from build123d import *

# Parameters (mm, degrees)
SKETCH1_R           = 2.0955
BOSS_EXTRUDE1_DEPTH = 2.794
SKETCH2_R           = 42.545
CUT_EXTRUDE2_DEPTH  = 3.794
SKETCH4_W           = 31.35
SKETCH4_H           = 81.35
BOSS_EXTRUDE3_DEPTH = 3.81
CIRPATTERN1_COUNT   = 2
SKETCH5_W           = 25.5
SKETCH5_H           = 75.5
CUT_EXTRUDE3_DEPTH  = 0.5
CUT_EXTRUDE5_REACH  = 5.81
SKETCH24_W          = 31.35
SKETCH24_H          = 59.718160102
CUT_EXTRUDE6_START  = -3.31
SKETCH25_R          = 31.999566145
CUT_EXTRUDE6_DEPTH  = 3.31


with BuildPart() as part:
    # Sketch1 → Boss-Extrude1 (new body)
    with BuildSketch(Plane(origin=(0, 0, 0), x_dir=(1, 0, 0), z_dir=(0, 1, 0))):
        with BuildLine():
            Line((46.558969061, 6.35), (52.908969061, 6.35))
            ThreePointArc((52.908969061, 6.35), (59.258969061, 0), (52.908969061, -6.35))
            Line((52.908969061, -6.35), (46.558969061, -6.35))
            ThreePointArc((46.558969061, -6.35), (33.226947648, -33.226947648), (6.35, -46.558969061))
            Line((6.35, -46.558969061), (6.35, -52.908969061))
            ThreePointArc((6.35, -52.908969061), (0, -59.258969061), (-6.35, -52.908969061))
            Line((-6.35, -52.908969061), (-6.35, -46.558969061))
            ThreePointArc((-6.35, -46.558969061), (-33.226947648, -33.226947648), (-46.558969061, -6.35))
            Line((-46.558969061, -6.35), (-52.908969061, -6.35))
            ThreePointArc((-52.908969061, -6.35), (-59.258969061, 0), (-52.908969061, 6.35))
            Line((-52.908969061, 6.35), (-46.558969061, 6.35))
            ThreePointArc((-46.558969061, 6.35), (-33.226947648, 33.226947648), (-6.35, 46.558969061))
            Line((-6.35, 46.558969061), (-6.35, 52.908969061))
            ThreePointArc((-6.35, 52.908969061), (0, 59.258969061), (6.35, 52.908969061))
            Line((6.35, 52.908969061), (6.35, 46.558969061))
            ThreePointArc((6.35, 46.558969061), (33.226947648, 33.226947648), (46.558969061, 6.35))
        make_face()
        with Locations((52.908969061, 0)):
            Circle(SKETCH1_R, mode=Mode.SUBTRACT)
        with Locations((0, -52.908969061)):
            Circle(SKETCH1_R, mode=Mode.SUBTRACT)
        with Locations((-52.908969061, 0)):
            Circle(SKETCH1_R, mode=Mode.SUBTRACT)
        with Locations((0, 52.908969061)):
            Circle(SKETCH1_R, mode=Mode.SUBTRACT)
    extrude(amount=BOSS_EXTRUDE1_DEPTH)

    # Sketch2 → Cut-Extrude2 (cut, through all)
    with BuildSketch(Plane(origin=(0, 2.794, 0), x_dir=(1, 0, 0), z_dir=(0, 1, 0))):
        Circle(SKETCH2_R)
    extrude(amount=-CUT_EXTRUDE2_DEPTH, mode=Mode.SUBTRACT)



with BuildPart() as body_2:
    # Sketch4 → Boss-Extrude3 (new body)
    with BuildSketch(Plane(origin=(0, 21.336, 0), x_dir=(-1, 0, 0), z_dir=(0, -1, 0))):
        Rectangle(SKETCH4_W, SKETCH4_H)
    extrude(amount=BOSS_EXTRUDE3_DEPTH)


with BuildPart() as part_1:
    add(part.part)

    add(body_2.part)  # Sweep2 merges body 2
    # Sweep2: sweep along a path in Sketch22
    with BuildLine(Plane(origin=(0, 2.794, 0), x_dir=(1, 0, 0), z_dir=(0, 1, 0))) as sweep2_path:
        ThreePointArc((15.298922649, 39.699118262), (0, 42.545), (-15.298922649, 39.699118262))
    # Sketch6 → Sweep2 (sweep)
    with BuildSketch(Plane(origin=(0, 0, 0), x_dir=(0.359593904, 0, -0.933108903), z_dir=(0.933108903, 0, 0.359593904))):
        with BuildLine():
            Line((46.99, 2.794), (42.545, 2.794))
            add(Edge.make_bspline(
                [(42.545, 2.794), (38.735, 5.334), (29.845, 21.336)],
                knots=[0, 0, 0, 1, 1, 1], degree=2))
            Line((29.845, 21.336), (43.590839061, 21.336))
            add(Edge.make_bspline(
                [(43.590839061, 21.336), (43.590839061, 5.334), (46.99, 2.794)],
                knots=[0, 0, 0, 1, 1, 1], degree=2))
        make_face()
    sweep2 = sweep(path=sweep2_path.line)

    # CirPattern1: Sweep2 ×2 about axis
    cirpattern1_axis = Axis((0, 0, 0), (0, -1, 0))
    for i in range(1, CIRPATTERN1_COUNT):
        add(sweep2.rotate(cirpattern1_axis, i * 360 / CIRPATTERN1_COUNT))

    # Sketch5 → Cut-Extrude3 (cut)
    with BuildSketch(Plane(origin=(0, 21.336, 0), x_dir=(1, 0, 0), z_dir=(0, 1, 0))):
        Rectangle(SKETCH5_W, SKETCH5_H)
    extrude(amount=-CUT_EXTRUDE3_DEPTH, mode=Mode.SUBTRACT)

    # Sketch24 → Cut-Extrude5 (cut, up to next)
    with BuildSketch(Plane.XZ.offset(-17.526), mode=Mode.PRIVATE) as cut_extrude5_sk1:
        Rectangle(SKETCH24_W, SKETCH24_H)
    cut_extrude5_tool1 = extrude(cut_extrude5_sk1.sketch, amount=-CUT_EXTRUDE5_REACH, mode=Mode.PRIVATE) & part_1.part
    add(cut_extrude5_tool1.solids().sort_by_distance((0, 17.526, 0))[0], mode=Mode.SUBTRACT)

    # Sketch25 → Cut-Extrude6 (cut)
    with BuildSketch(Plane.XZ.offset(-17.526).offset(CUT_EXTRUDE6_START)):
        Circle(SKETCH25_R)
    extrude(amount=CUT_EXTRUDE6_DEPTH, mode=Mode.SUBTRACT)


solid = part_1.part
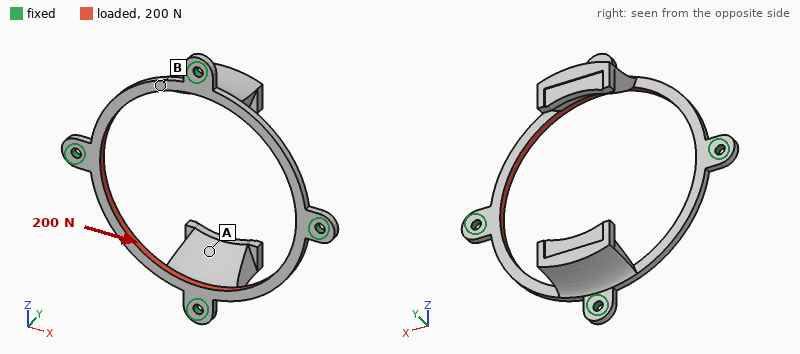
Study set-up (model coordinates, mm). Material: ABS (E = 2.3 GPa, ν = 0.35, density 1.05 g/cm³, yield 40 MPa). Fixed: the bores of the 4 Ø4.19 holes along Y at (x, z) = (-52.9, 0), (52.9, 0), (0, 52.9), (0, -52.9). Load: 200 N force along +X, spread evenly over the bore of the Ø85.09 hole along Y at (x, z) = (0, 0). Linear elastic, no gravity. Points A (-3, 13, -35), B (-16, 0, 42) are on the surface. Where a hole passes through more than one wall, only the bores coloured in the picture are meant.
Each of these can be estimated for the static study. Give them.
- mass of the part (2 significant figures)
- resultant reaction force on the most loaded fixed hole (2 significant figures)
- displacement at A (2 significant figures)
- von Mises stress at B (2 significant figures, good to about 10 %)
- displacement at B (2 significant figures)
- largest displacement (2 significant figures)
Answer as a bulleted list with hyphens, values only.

- 15 g
- 81 N
- 0.073 mm
- 2.7 MPa
- 0.066 mm
- 0.11 mm
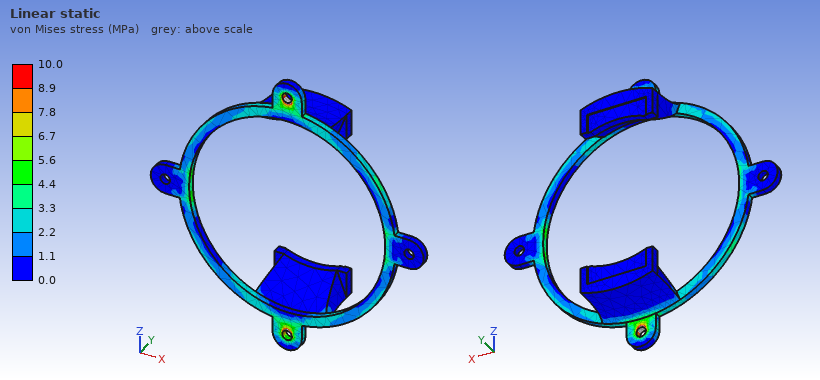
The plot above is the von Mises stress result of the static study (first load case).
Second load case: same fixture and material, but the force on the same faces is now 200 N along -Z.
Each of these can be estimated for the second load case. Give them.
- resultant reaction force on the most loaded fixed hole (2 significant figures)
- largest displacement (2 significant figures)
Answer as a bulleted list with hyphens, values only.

- 72 N
- 0.10 mm
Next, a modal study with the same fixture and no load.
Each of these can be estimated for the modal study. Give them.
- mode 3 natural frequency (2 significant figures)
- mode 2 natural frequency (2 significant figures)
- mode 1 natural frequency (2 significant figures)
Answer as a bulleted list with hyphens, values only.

- 560 Hz
- 430 Hz
- 420 Hz
